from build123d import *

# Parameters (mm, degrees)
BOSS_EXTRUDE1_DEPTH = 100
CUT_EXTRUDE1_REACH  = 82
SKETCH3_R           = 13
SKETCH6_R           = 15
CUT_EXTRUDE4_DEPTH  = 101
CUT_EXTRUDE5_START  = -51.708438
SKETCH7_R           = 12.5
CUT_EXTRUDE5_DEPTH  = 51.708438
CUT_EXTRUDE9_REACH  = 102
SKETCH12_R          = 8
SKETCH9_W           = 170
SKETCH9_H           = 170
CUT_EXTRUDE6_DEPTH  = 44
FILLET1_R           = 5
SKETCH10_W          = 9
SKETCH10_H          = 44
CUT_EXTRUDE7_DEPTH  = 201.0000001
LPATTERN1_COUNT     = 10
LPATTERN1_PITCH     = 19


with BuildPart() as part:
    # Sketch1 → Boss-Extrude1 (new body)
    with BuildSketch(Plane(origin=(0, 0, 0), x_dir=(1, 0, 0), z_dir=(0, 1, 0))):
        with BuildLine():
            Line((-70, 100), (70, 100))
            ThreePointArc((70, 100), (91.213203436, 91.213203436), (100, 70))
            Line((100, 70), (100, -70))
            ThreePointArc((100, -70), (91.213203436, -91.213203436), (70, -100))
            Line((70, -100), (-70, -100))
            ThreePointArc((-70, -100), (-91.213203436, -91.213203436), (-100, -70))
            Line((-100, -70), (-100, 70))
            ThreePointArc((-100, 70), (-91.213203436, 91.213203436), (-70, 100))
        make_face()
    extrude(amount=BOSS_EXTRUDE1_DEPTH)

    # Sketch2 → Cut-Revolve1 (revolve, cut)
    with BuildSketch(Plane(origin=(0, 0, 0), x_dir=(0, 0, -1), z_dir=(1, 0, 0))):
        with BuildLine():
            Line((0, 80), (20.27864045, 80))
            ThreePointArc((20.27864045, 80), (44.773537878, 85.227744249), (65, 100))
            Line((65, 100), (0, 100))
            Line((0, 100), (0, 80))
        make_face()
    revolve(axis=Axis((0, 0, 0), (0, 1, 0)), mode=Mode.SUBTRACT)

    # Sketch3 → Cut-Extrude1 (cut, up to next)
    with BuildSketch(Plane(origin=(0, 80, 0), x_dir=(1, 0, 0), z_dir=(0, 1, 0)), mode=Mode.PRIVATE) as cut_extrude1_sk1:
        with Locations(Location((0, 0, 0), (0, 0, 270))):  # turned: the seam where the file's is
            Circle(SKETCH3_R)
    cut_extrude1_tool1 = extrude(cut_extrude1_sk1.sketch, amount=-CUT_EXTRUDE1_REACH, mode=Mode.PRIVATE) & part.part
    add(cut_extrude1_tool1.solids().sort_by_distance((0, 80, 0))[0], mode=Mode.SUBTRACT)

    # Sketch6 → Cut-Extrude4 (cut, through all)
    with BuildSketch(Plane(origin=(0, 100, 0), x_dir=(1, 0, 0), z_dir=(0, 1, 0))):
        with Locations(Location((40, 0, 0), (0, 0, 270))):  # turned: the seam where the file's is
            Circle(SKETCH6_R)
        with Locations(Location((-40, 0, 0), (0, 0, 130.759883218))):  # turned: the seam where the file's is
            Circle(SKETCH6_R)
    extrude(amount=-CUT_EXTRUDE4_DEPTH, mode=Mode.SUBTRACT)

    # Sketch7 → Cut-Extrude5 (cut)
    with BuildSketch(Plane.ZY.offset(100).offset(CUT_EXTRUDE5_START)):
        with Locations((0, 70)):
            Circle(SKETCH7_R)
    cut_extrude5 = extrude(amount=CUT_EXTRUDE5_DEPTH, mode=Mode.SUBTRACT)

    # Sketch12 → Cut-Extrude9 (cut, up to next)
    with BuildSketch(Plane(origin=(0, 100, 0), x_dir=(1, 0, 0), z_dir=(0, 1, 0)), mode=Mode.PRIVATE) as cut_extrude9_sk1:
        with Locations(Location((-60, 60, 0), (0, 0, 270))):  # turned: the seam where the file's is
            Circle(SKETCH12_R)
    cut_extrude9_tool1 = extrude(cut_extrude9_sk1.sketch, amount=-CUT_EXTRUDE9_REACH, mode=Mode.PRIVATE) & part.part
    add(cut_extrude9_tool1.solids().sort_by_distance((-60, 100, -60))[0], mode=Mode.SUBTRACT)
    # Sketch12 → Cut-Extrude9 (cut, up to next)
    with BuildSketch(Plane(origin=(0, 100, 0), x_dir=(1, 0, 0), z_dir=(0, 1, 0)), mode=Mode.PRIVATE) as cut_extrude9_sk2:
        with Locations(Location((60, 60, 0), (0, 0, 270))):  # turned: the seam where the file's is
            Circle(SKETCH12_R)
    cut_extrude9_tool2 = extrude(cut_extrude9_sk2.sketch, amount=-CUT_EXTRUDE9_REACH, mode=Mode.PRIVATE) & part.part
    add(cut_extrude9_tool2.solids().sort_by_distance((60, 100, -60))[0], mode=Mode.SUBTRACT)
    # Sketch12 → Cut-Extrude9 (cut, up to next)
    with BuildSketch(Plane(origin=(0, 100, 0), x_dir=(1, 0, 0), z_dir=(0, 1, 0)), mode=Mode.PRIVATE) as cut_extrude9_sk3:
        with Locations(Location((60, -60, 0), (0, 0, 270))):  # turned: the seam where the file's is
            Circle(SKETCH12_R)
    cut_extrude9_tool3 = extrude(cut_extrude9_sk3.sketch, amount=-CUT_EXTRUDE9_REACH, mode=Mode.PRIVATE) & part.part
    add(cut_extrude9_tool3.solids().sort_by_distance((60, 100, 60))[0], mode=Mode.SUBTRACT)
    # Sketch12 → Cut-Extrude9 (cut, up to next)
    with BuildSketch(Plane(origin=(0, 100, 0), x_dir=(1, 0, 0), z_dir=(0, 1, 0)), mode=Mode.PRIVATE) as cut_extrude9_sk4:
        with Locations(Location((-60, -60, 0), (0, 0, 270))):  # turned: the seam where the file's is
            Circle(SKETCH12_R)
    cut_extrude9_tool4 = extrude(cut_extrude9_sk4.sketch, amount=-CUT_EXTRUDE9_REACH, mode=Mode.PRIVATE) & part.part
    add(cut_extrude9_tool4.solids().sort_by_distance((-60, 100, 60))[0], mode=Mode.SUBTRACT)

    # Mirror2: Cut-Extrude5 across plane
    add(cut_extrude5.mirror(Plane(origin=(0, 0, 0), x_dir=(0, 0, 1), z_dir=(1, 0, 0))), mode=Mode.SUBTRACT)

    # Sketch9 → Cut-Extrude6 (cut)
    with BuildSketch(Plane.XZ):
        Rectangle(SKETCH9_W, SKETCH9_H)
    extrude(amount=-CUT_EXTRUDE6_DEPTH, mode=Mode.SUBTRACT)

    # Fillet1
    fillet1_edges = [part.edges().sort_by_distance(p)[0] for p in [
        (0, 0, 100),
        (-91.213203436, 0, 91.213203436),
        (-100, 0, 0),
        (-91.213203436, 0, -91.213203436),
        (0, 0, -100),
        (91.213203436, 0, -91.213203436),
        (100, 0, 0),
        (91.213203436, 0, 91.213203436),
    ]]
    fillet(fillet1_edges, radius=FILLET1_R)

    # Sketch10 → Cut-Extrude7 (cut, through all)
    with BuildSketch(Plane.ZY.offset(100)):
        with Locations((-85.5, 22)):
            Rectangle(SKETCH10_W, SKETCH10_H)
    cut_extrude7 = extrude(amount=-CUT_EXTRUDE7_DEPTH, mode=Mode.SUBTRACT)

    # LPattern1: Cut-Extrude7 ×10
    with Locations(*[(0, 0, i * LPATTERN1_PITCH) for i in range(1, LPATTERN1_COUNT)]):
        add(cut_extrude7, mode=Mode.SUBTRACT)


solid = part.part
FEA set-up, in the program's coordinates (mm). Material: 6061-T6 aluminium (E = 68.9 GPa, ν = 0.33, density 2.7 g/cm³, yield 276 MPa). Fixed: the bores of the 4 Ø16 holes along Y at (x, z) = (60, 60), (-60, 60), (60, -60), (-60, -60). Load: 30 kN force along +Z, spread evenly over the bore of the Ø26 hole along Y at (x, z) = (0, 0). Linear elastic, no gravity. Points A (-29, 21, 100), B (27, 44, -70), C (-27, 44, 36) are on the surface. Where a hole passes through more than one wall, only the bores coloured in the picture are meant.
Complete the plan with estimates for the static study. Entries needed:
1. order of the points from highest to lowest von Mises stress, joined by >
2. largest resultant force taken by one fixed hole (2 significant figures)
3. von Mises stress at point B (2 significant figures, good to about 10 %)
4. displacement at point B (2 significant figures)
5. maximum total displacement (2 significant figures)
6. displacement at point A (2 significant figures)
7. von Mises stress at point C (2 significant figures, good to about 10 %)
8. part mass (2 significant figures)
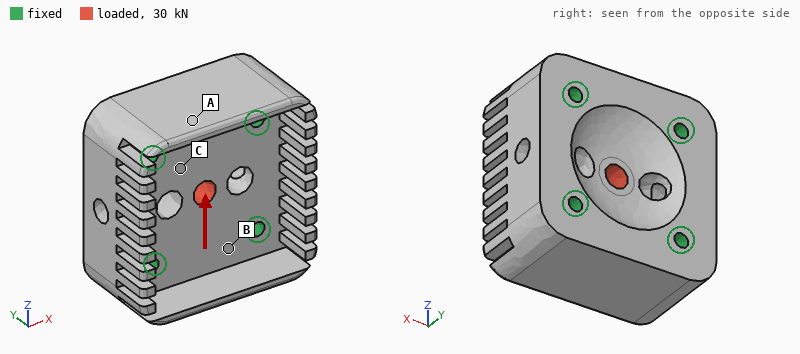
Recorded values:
C > B > A
7.9 kN
3.1 MPa
3.0 µm
8.1 µm
3.1 µm
5.4 MPa
5.7 kg
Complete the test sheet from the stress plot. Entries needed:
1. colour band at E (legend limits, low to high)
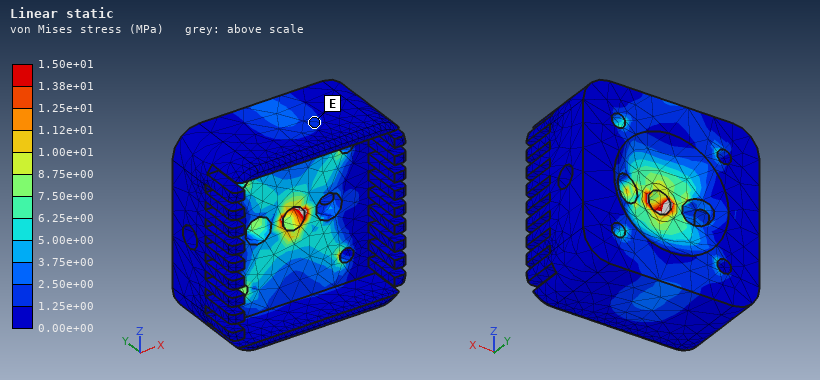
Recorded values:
1.25e+00 to 2.50e+00 MPa
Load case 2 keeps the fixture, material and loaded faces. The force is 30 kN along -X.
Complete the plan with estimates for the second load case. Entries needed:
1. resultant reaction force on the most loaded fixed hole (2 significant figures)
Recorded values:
8.6 kN
